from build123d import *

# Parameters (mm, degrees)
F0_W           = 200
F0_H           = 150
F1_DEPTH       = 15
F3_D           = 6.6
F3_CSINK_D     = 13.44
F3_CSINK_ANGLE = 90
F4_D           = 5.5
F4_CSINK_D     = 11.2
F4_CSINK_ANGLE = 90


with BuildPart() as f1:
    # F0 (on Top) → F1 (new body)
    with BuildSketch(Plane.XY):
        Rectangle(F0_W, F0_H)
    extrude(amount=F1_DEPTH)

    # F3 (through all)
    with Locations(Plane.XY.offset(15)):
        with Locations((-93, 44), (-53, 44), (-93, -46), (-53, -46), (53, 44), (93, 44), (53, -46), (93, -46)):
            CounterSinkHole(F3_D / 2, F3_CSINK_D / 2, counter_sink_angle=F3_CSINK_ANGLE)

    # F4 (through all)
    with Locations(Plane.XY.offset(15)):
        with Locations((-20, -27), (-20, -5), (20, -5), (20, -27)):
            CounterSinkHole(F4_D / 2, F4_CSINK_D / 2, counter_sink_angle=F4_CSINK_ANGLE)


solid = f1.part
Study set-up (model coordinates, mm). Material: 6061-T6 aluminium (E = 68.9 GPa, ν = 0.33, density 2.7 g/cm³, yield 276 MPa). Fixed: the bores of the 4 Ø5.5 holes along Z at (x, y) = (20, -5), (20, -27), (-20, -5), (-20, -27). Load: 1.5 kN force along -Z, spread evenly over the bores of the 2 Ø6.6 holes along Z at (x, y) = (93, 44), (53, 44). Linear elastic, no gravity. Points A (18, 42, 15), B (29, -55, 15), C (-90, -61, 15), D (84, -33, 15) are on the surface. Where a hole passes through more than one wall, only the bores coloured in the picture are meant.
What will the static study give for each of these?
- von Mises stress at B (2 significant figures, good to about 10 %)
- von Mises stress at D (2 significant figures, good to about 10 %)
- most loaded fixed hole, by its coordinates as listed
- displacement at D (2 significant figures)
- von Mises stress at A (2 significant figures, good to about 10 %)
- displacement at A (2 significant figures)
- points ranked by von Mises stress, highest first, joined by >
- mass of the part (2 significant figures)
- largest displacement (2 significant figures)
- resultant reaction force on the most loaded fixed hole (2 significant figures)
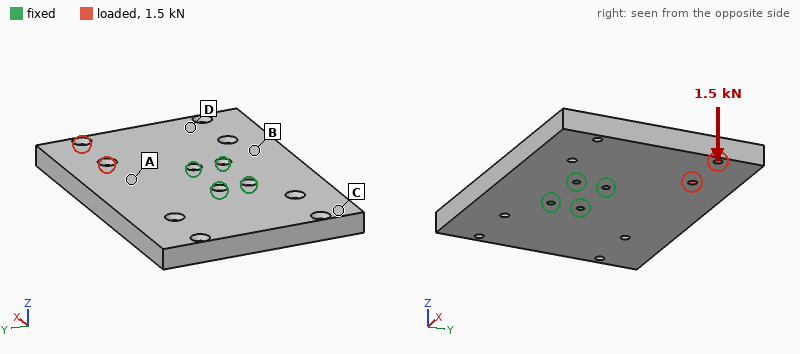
6.4 MPa
8.9 MPa
(20, -5)
0.036 mm
12 MPa
0.043 mm
A > D > B > C
1.2 kg
0.21 mm
3.2 kN
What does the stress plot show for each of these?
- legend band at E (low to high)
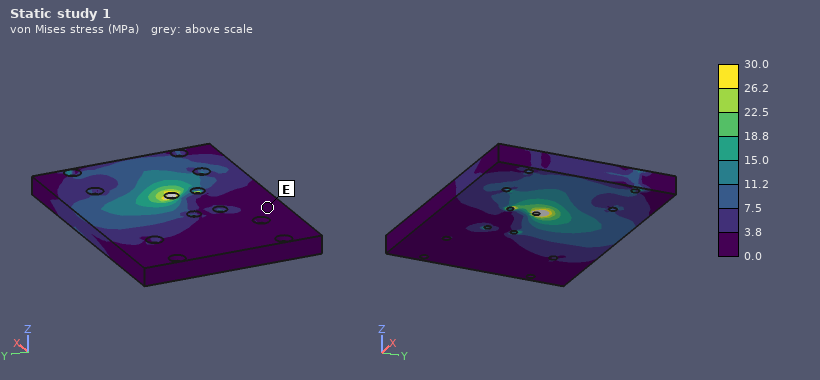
0.0 to 3.8 MPa
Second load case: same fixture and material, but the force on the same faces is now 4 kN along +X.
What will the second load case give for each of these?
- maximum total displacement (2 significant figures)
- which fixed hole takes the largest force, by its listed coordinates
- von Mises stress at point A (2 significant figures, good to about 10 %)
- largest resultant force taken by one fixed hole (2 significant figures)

26 µm
(20, -5)
3.1 MPa
3.7 kN
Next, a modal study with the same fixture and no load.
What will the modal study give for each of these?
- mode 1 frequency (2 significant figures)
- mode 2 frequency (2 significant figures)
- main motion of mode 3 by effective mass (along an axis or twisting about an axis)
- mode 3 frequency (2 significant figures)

1200 Hz
1200 Hz
along Z
1700 Hz
